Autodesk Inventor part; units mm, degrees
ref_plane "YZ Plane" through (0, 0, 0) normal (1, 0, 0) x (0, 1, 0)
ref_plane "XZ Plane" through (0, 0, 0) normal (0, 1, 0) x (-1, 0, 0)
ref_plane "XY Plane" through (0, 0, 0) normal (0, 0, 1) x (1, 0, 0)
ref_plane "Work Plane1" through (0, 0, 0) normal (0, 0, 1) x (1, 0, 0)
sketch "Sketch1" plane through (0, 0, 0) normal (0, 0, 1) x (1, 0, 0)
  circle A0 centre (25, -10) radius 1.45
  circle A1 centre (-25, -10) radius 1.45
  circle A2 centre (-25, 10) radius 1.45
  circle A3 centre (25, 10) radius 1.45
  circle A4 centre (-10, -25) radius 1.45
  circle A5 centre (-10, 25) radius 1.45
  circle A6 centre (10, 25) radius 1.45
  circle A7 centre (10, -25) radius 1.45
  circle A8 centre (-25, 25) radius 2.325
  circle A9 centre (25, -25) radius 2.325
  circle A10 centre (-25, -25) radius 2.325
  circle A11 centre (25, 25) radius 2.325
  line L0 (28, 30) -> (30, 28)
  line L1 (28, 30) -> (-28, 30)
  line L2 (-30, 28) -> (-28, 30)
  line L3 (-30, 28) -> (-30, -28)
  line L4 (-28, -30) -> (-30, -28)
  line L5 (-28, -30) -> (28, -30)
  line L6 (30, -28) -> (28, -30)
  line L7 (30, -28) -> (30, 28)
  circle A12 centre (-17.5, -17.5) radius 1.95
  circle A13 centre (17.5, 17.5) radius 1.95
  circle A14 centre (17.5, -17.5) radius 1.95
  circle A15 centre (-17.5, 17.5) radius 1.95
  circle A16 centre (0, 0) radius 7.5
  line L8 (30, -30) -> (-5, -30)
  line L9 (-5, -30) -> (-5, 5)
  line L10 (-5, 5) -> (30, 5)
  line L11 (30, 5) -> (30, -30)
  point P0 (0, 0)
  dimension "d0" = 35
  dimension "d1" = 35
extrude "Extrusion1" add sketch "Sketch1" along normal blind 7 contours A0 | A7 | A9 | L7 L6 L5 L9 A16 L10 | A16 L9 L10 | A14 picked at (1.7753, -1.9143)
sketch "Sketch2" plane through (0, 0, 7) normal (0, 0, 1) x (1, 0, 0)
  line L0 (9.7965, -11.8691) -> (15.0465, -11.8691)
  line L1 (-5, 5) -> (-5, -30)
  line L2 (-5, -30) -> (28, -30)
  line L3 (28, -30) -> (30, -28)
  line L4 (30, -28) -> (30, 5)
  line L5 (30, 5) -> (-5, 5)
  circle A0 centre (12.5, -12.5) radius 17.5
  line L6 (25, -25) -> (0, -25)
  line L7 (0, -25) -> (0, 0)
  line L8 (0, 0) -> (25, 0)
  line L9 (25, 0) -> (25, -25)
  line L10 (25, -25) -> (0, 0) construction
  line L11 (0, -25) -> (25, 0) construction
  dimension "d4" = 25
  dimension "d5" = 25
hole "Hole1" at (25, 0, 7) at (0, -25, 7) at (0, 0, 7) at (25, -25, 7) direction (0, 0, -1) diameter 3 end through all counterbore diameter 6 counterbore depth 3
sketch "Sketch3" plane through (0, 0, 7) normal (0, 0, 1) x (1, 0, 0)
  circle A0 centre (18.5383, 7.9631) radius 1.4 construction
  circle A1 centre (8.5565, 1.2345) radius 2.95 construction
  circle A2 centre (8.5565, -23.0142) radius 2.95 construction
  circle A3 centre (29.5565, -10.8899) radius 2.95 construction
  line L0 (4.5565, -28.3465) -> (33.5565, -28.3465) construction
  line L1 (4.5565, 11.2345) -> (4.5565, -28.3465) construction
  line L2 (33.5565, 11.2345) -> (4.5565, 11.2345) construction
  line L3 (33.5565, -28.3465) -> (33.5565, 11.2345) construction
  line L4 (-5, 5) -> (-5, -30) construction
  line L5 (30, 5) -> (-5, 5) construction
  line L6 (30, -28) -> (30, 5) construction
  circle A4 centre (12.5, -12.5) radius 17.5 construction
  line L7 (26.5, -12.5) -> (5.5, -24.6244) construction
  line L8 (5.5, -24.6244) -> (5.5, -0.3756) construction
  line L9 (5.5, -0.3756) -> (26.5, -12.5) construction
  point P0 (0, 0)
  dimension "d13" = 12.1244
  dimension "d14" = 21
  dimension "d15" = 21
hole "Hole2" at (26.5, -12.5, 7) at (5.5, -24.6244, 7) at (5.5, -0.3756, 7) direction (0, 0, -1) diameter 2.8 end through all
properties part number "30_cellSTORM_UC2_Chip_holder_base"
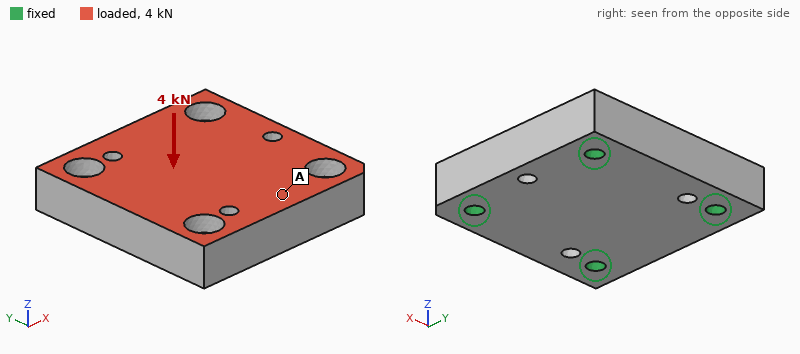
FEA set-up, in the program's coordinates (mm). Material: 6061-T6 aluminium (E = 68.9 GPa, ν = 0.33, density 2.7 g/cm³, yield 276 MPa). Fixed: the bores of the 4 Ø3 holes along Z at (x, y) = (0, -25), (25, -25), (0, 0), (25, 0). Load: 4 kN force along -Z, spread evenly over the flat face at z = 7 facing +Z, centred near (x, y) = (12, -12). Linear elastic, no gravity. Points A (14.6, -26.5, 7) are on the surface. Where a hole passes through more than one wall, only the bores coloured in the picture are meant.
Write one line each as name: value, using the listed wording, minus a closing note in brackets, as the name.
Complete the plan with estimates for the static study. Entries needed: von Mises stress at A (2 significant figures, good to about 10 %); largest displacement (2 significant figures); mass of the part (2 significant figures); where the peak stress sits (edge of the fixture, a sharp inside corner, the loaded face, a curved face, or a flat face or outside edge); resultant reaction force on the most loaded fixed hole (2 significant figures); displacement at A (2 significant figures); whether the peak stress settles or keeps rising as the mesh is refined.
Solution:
von Mises stress at A: 19 MPa
largest displacement: 9.9 µm
mass of the part: 22 g
where the peak stress sits: edge of the fixture
resultant reaction force on the most loaded fixed hole: 1.1 kN
displacement at A: 6.5 µm
whether the peak stress settles or keeps rising as the mesh is refined: keeps rising
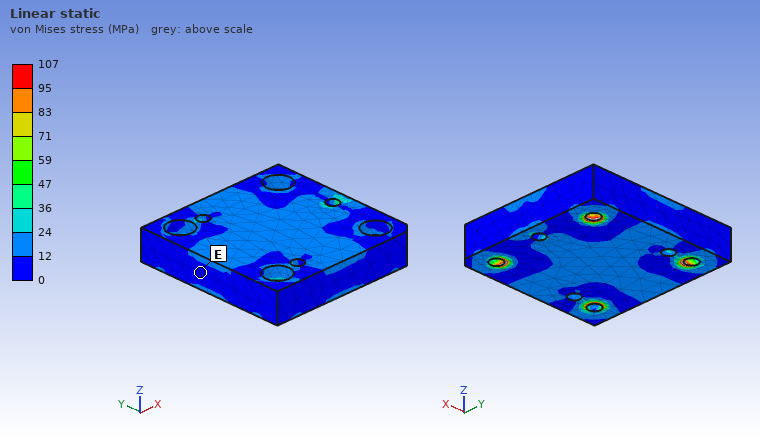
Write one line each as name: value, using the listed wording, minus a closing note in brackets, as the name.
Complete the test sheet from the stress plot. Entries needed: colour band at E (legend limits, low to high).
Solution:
colour band at E: 0 to 12 MPa
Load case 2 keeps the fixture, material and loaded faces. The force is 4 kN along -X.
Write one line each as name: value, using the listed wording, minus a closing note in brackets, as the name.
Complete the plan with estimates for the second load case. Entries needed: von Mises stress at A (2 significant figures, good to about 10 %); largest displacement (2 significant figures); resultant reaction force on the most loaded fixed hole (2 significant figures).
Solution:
von Mises stress at A: 8.7 MPa
largest displacement: 7.2 µm
resultant reaction force on the most loaded fixed hole: 1.1 kN
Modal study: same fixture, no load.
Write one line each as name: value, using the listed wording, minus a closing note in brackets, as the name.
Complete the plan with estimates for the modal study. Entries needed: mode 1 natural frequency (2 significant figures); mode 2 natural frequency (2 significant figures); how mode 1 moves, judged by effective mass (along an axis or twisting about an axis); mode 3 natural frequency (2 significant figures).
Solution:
mode 1 natural frequency: 25 kHz
mode 2 natural frequency: 35 kHz
how mode 1 moves, judged by effective mass: along Z
mode 3 natural frequency: 36 kHz
